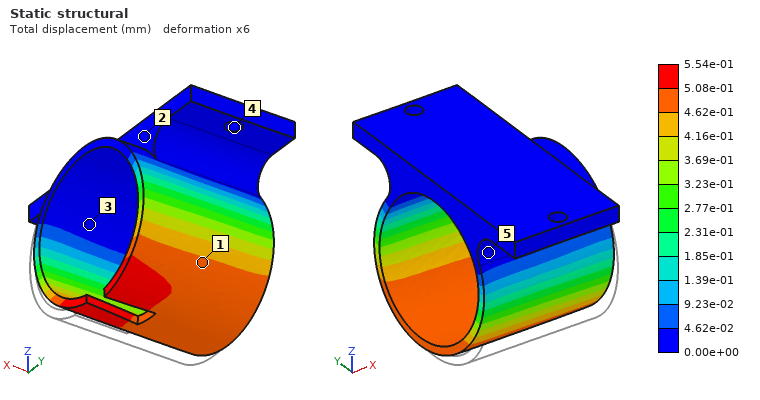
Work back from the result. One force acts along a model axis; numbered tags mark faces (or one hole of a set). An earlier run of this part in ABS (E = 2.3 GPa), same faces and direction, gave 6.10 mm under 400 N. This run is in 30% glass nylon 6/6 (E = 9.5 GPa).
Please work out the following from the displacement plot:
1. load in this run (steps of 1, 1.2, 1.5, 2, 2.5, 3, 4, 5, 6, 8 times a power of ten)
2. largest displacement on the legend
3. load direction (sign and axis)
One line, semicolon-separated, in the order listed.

150 N; 5.54e-01 mm; +Y
